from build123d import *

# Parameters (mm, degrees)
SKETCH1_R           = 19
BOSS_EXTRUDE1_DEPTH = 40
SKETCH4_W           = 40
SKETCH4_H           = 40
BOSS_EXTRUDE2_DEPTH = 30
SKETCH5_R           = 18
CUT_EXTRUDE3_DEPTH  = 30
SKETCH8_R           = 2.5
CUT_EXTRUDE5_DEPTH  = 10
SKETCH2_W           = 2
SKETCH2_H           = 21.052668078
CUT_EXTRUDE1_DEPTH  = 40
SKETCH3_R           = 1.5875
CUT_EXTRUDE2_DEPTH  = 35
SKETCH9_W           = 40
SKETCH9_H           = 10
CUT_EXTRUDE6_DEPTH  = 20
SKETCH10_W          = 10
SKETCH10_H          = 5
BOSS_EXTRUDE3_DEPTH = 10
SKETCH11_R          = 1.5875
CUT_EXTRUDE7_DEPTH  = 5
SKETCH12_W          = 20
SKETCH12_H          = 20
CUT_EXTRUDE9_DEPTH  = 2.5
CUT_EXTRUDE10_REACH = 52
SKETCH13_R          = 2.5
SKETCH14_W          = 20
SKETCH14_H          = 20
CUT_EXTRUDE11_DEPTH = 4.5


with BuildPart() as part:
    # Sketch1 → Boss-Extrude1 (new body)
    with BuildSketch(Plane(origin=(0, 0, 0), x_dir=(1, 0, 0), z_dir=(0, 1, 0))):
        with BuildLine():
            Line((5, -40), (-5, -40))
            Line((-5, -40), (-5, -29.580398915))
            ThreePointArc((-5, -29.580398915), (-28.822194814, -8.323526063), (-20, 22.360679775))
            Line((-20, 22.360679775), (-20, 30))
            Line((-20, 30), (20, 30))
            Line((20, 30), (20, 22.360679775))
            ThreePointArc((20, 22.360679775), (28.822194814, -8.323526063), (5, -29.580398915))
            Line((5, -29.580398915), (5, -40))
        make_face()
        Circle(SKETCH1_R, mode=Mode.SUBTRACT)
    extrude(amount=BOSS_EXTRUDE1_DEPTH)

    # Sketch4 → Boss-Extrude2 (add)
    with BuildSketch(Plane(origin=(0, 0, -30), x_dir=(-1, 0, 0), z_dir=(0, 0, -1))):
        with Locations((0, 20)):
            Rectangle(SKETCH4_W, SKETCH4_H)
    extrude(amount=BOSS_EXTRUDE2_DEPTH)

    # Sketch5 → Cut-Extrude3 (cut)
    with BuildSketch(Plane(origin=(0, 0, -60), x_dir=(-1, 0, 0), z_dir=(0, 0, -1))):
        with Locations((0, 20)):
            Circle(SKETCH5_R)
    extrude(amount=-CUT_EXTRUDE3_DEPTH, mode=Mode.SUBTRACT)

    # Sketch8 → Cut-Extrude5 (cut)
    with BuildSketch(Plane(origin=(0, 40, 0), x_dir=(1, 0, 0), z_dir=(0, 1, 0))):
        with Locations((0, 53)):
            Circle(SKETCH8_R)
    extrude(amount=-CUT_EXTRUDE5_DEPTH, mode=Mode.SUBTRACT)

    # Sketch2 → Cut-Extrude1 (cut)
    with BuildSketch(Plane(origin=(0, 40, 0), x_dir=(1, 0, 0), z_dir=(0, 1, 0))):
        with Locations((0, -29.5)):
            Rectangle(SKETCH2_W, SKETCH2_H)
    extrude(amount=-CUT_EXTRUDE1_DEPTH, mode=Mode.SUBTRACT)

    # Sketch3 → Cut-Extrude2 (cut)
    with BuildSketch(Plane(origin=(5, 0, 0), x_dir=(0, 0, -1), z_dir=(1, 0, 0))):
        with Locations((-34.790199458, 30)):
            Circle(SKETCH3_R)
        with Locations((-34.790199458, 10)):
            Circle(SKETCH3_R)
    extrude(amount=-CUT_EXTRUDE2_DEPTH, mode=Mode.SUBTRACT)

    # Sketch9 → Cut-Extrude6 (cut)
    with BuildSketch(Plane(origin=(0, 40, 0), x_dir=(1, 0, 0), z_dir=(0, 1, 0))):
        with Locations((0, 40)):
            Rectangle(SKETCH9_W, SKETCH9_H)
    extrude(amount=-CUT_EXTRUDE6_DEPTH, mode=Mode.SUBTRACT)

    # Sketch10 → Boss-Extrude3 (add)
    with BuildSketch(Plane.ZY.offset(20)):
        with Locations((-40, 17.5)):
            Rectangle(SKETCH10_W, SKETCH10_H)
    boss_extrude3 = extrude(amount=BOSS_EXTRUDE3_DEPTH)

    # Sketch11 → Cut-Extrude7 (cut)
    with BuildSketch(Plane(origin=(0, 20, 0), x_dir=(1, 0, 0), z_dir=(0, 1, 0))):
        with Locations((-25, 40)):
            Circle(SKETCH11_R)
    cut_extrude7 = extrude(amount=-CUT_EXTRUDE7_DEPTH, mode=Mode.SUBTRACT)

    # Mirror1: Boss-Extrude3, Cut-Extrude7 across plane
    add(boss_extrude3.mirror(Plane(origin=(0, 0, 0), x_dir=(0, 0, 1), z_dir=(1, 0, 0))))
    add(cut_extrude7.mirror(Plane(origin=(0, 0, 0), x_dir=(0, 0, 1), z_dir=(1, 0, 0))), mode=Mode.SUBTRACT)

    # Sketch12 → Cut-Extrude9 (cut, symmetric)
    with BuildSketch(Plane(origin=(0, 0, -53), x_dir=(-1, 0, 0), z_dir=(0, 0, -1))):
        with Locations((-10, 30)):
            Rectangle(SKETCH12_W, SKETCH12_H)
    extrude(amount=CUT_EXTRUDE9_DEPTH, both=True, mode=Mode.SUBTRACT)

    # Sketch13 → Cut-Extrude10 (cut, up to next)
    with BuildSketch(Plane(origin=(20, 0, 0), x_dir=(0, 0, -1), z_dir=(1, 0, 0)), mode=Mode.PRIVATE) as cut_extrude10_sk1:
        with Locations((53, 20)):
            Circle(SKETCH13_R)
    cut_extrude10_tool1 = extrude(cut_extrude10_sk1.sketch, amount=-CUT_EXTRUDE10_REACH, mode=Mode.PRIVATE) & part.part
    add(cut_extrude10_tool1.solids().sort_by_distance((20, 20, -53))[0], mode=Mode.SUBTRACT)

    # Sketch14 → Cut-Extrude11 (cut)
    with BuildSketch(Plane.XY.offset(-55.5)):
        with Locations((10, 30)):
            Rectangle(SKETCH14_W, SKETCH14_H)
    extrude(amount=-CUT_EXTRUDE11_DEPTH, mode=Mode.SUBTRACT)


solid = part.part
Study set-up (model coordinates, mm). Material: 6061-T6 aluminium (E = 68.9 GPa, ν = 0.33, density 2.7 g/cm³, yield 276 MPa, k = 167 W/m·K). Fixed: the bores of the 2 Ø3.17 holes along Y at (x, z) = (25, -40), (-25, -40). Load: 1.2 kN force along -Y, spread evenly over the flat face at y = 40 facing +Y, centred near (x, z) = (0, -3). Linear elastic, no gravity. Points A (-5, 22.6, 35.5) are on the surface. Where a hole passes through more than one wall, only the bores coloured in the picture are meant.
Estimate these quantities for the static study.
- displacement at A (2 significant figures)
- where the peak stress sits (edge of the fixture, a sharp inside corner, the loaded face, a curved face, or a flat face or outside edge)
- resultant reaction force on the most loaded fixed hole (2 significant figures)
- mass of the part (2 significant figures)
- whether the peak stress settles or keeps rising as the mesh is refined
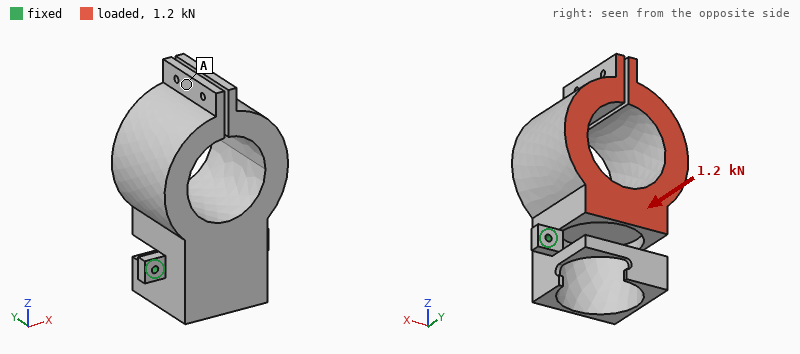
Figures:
1.3 mm
edge of the fixture
620 N
240 g
keeps rising
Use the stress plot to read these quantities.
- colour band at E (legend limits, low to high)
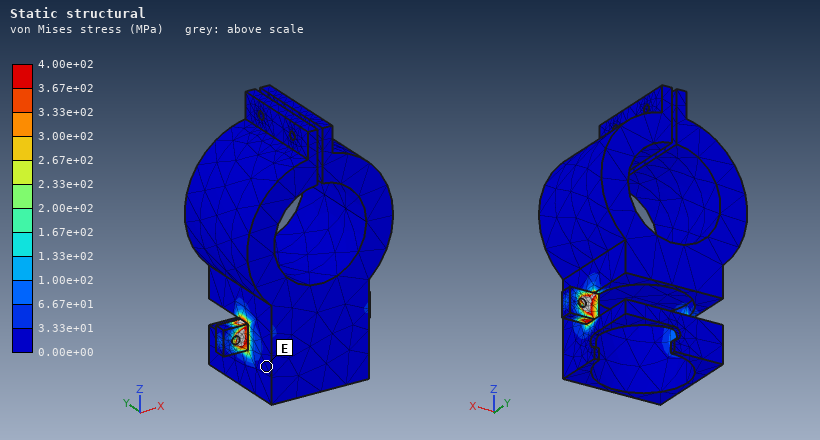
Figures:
0.00e+00 to 3.33e+01 MPa
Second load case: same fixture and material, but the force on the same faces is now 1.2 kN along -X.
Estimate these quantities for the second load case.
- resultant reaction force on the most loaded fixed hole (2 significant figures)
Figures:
1.3 kN
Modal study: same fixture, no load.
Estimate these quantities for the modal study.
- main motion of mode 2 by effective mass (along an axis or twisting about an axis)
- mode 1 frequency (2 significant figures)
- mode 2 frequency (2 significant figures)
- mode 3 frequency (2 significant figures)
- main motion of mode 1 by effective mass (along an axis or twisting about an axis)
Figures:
along X
390 Hz
1500 Hz
2000 Hz
along Y
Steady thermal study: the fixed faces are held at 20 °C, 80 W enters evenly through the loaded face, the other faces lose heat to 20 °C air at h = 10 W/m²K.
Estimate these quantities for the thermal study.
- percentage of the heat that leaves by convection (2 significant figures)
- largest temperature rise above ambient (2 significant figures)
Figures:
16 %
72 K
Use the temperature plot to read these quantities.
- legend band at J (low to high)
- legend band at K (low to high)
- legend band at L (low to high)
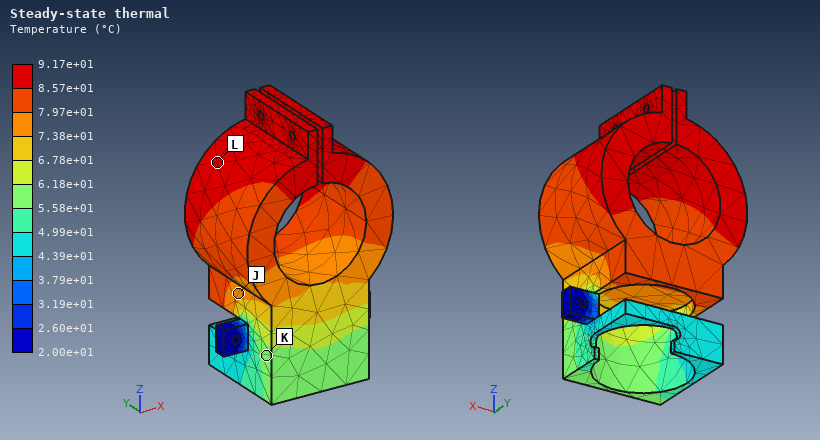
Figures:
7.38e+01 to 7.97e+01 °C
5.58e+01 to 6.18e+01 °C
8.57e+01 to 9.17e+01 °C
